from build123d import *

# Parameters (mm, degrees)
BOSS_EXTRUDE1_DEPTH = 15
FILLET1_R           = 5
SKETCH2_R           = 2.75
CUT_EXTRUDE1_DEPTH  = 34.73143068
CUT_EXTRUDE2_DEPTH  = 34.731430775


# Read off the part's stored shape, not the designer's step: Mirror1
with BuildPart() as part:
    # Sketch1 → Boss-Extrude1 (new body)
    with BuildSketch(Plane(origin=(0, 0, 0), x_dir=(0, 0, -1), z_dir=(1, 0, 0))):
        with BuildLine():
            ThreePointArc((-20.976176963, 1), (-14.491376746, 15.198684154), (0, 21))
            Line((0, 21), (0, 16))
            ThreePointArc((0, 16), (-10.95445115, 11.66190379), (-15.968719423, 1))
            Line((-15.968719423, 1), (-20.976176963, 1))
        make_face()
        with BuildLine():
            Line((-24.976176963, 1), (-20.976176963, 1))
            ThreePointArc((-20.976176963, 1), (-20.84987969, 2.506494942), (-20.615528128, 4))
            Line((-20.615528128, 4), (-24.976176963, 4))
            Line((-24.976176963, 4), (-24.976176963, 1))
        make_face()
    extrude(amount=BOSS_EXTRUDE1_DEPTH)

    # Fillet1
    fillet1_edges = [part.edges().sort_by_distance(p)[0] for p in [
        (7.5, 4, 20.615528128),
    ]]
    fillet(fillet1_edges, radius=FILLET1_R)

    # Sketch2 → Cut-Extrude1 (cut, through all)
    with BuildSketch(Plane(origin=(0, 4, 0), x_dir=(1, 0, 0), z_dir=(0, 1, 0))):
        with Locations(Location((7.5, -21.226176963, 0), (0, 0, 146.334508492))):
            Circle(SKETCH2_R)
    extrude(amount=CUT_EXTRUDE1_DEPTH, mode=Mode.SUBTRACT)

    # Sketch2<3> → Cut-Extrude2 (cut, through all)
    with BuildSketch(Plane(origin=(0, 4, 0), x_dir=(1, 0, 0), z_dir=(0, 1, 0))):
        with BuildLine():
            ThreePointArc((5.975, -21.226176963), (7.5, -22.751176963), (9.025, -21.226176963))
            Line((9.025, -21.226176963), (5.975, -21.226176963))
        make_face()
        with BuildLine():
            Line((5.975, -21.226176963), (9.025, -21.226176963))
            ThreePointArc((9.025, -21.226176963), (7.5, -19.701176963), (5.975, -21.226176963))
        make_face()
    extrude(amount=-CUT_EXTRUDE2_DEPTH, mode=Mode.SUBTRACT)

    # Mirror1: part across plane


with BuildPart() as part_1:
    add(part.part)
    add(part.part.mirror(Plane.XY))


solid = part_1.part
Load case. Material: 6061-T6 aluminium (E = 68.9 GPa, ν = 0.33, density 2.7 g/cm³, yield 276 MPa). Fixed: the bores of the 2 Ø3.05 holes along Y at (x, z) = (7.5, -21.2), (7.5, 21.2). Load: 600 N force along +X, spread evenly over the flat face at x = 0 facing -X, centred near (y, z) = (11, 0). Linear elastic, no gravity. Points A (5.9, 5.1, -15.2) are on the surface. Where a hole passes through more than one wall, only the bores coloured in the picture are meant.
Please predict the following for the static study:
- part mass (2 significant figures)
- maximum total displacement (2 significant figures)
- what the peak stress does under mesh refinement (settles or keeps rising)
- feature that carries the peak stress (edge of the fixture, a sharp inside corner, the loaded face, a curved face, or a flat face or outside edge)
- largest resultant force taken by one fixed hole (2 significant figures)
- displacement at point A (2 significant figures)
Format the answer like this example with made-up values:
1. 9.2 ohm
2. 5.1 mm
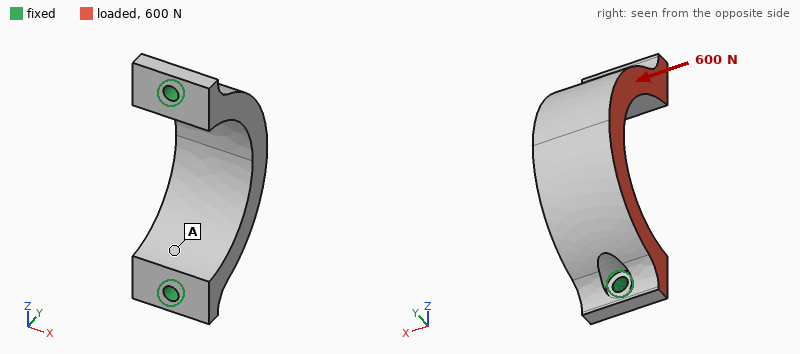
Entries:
1. 12 g
2. 50 µm
3. keeps rising
4. edge of the fixture
5. 300 N
6. 9.5 µm
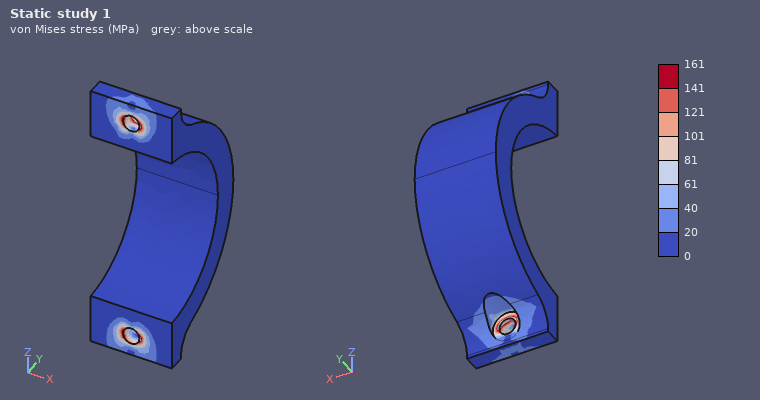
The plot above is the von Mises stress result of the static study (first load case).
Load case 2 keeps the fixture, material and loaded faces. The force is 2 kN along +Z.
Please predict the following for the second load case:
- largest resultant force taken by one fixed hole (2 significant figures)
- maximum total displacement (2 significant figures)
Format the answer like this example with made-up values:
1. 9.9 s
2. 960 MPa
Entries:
1. 1.1 kN
2. 49 µm
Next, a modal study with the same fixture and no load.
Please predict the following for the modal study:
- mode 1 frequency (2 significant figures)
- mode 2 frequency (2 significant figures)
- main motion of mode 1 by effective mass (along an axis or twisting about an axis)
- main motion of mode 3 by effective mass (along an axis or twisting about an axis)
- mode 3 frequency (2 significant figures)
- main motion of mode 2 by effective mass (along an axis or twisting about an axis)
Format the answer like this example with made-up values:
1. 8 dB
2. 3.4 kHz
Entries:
1. 5800 Hz
2. 13 kHz
3. along X
4. twisting about Y
5. 17 kHz
6. along Z
